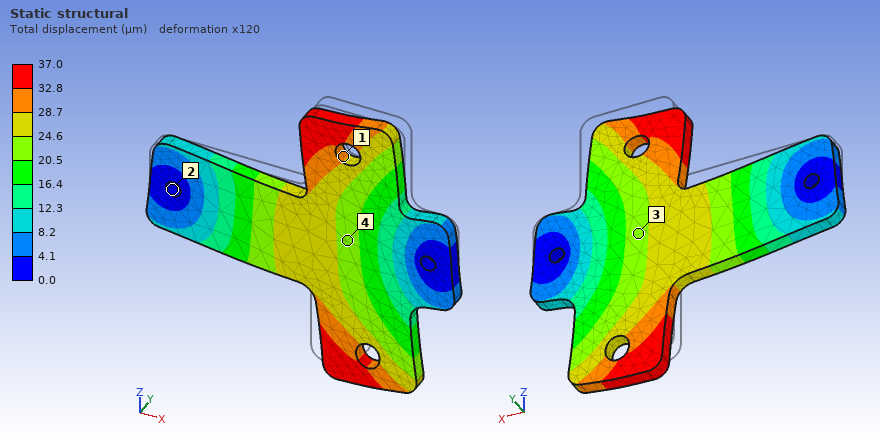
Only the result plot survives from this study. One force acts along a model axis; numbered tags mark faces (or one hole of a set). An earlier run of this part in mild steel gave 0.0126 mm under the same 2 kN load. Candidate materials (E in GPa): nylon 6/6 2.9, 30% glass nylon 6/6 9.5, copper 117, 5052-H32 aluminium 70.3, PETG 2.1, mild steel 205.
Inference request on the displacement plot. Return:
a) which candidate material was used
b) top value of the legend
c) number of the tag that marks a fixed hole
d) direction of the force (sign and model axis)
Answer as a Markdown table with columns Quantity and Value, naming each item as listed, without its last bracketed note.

| Quantity | Value |
|---|---|
| which candidate material was used | 5052-H32 aluminium |
| top value of the legend | 37.0 µm |
| number of the tag that marks a fixed hole | 2 |
| direction of the force | -Z |
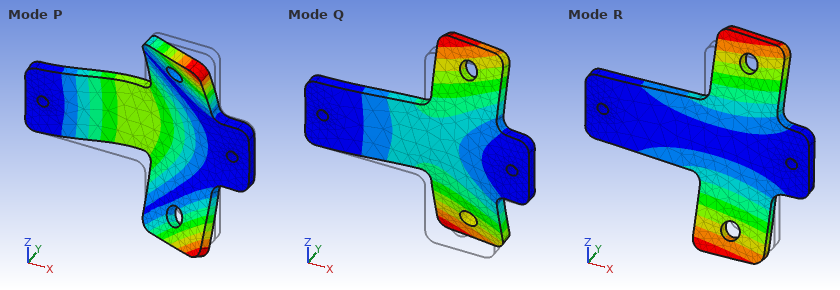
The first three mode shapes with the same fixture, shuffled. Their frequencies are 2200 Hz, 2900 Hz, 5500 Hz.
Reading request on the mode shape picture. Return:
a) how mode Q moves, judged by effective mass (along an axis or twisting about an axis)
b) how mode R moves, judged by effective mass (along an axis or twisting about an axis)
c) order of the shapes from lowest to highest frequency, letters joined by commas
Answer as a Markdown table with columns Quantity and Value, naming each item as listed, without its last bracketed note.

| Quantity | Value |
|---|---|
| how mode Q moves, judged by effective mass | along Y |
| how mode R moves, judged by effective mass | twisting about X |
| order of the shapes from lowest to highest frequency, letters joined by commas | R, Q, P |
